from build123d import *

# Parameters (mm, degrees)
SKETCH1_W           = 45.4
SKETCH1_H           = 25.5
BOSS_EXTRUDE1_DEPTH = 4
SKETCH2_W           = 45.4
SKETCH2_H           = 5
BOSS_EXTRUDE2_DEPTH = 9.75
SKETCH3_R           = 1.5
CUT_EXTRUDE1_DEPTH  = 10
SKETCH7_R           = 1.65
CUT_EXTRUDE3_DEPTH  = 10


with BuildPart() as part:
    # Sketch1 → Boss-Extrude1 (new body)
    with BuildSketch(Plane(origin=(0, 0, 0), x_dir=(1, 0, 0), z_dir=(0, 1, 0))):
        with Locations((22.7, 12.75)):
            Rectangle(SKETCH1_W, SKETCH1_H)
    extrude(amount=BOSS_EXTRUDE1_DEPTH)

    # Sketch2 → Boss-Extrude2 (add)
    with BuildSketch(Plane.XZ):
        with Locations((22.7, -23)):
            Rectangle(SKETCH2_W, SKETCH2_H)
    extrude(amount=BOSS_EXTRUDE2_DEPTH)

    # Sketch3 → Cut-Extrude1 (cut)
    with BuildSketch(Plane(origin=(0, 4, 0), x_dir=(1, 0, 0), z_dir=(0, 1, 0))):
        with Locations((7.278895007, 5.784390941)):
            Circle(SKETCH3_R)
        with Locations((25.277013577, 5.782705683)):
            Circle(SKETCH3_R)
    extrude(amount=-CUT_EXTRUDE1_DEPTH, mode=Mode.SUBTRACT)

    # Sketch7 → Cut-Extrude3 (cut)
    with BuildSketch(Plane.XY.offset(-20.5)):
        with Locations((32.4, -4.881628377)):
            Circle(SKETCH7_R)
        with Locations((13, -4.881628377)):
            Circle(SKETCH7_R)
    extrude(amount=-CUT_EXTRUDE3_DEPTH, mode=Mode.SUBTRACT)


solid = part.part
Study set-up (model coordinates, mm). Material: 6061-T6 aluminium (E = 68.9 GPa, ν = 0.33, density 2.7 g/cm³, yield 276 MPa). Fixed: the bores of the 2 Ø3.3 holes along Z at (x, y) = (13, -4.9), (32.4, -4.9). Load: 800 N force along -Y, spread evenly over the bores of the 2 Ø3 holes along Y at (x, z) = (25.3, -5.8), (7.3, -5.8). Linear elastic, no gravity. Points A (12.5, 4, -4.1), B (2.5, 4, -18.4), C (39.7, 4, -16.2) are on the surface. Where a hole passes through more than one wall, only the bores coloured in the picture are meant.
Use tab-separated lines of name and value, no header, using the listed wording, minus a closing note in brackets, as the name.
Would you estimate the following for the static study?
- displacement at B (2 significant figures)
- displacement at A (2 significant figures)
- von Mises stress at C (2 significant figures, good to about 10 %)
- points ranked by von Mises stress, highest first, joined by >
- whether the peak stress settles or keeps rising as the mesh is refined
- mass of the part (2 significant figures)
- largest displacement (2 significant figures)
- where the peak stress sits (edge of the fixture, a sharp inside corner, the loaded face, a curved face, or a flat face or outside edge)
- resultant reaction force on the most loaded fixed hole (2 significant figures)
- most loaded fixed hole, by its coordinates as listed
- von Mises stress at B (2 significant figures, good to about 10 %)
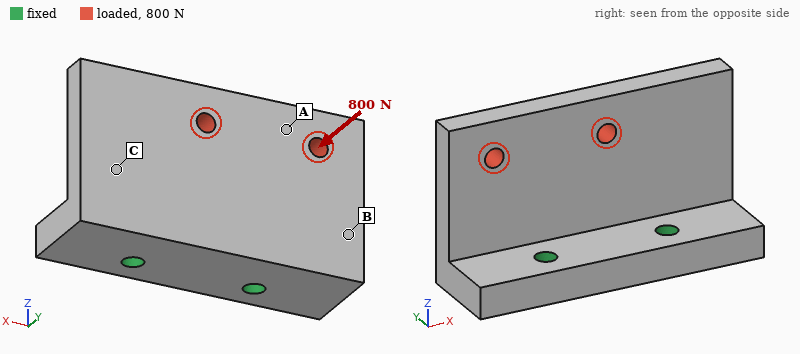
displacement at B	0.044 mm
displacement at A	0.17 mm
von Mises stress at C	53 MPa
points ranked by von Mises stress, highest first, joined by >	B > C > A
whether the peak stress settles or keeps rising as the mesh is refined	keeps rising
mass of the part	18 g
largest displacement	0.23 mm
where the peak stress sits	edge of the fixture
resultant reaction force on the most loaded fixed hole	630 N
most loaded fixed hole, by its coordinates as listed	(13, -4.9)
von Mises stress at B	86 MPa
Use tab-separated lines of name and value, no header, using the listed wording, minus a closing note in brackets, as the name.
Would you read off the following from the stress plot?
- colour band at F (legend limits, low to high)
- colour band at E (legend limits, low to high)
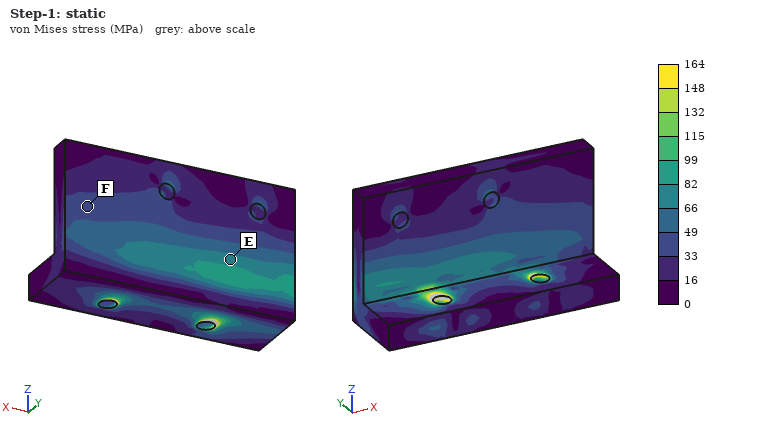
colour band at F	33 to 49 MPa
colour band at E	66 to 82 MPa
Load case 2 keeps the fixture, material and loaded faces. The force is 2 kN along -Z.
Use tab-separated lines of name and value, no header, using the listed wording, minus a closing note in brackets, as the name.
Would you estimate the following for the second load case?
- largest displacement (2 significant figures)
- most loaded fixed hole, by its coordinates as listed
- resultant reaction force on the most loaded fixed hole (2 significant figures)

largest displacement	80 µm
most loaded fixed hole, by its coordinates as listed	(13, -4.9)
resultant reaction force on the most loaded fixed hole	1.5 kN
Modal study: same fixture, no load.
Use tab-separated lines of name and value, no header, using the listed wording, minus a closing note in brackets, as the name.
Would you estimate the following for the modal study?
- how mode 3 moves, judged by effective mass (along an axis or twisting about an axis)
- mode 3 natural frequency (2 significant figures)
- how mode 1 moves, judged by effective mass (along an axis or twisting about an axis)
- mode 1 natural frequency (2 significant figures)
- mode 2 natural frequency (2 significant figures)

how mode 3 moves, judged by effective mass	along X
mode 3 natural frequency	12 kHz
how mode 1 moves, judged by effective mass	along Y
mode 1 natural frequency	4900 Hz
mode 2 natural frequency	7600 Hz
